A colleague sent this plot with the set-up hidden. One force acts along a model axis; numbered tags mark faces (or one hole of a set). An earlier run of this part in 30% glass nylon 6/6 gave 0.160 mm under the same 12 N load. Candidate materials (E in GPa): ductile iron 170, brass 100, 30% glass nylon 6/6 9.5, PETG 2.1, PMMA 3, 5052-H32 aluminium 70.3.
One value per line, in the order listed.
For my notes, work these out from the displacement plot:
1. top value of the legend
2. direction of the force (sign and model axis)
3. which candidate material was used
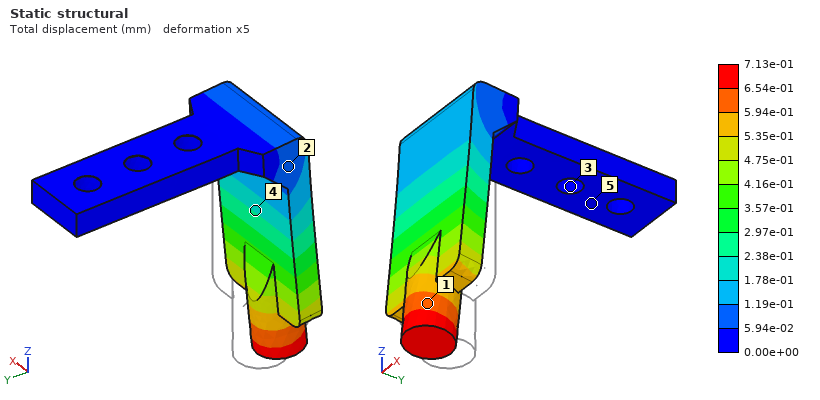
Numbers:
7.13e-01 mm
-Y
PETG
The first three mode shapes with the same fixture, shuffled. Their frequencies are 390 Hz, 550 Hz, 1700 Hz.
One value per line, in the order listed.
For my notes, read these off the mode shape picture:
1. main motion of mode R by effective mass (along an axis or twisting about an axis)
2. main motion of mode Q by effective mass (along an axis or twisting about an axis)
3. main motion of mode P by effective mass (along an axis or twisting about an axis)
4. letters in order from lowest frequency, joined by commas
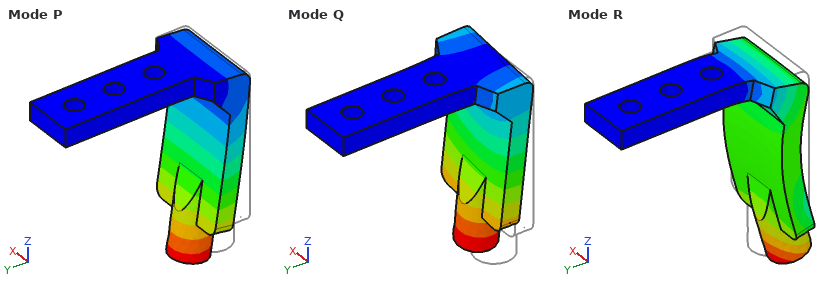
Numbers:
along Z
along X
along Y
P, Q, R
